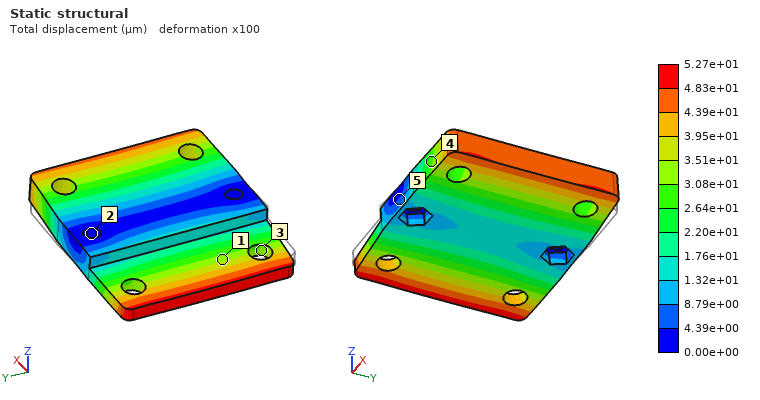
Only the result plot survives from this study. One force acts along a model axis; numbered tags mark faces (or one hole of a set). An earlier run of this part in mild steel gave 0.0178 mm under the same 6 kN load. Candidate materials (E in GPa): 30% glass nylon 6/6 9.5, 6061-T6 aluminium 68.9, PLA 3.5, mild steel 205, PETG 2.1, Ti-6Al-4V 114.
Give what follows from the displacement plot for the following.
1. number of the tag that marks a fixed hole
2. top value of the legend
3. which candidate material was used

2
5.27e+01 µm
6061-T6 aluminium
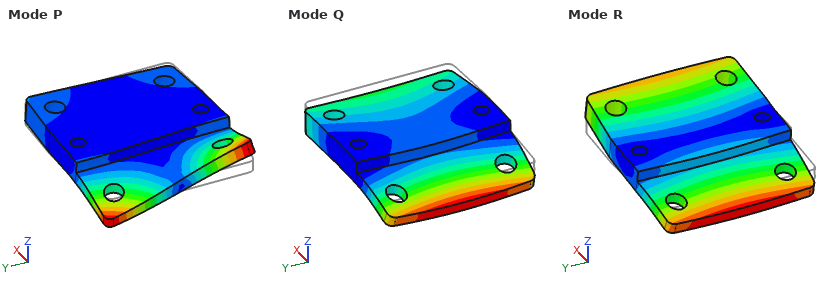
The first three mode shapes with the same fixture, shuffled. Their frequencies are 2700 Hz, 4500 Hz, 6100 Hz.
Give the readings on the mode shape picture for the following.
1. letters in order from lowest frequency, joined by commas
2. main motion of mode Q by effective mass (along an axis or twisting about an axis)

R, Q, P
along Z
